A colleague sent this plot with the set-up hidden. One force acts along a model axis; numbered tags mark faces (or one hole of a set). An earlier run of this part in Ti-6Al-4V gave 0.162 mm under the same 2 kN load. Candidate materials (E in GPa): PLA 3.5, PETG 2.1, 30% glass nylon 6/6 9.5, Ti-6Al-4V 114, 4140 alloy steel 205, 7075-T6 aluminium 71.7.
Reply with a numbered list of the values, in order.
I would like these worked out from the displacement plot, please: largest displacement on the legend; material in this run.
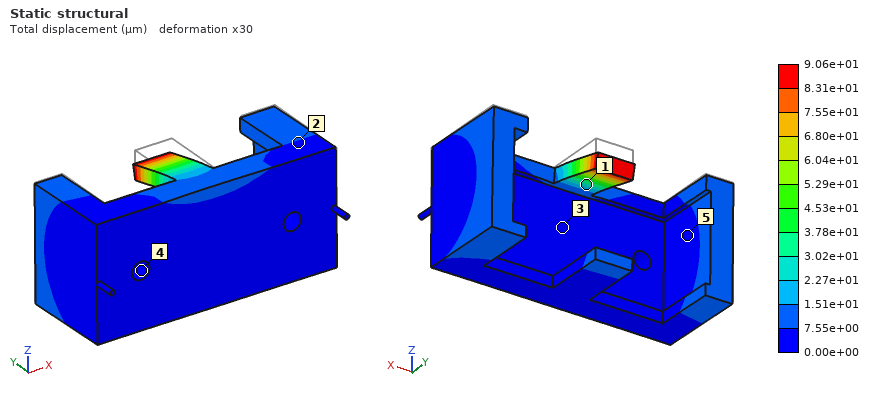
1. 9.06e+01 µm
2. 4140 alloy steel
